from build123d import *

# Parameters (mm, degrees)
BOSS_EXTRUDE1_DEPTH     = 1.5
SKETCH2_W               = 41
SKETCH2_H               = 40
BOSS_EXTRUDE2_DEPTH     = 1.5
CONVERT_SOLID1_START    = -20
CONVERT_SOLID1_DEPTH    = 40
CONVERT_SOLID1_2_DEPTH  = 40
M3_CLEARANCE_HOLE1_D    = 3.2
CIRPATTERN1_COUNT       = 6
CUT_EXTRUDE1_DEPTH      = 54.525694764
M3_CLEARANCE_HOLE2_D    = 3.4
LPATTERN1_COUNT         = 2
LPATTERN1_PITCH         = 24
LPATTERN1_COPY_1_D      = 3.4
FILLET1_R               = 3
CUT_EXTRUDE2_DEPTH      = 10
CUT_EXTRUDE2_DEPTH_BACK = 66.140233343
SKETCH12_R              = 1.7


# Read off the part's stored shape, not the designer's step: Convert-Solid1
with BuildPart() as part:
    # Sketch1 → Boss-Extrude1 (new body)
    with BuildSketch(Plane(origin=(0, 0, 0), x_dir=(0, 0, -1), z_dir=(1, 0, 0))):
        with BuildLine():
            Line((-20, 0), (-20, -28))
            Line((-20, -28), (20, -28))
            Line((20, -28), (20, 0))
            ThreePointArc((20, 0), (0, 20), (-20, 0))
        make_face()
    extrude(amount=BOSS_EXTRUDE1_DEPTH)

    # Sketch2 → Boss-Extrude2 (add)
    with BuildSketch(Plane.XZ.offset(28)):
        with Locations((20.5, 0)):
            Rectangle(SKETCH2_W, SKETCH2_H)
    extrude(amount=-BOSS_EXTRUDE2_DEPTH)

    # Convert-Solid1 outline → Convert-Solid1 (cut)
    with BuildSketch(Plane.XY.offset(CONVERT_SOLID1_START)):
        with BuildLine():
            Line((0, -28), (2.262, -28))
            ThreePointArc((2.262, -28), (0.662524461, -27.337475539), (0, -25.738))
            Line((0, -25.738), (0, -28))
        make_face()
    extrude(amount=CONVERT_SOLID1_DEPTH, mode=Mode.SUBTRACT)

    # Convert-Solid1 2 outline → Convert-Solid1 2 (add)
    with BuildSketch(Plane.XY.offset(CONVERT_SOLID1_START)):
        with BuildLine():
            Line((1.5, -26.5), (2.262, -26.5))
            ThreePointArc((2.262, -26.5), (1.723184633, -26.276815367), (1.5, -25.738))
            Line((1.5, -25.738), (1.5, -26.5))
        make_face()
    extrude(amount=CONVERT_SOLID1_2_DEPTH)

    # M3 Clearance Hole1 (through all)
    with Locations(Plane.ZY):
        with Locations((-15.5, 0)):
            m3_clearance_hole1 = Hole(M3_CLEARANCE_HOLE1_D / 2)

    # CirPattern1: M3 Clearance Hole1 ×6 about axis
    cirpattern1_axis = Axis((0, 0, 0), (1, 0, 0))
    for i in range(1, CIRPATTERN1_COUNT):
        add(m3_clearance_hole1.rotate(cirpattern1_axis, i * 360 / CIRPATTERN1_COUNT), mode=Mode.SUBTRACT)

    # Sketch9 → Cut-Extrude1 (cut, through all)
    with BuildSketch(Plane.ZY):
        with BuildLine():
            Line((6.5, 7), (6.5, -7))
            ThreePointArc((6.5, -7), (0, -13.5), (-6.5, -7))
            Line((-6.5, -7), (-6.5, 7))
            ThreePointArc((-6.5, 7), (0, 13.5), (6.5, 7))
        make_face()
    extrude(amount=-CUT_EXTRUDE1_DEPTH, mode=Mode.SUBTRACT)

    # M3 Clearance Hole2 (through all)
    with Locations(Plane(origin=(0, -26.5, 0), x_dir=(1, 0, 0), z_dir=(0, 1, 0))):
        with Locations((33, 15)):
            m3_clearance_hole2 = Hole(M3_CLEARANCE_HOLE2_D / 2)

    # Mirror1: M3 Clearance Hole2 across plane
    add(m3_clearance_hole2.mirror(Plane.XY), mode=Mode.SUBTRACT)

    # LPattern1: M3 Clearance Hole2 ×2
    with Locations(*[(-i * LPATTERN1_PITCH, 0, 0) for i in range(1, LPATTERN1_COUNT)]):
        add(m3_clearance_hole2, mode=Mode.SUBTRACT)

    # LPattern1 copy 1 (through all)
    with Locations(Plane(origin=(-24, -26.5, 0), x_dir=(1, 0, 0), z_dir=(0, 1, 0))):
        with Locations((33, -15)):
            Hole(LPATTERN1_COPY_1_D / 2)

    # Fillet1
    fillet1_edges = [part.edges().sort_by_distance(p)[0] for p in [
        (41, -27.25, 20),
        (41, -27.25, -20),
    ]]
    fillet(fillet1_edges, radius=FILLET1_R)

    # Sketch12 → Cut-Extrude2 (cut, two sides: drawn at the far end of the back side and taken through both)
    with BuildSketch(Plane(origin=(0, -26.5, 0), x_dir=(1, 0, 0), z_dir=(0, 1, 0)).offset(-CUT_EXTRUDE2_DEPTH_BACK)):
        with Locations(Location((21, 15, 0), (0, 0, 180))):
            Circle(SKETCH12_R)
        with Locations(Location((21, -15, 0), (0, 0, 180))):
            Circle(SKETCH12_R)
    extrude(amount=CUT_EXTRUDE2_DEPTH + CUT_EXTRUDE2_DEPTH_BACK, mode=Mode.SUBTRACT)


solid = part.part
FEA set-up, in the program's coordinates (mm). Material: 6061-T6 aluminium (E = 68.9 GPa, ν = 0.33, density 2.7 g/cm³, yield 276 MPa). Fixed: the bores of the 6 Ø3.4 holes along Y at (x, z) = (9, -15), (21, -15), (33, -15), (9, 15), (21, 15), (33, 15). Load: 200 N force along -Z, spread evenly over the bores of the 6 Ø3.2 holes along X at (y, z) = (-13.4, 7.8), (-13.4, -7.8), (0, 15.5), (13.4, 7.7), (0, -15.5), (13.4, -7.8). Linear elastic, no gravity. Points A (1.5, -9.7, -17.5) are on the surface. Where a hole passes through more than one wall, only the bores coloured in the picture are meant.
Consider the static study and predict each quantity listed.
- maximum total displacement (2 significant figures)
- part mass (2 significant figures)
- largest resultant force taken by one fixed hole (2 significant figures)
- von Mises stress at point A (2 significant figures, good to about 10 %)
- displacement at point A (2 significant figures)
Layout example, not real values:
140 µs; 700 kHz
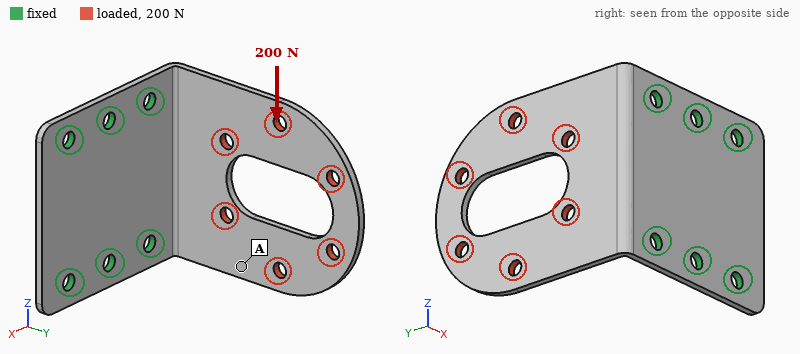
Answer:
0.24 mm; 12 g; 210 N; 22 MPa; 0.16 mm
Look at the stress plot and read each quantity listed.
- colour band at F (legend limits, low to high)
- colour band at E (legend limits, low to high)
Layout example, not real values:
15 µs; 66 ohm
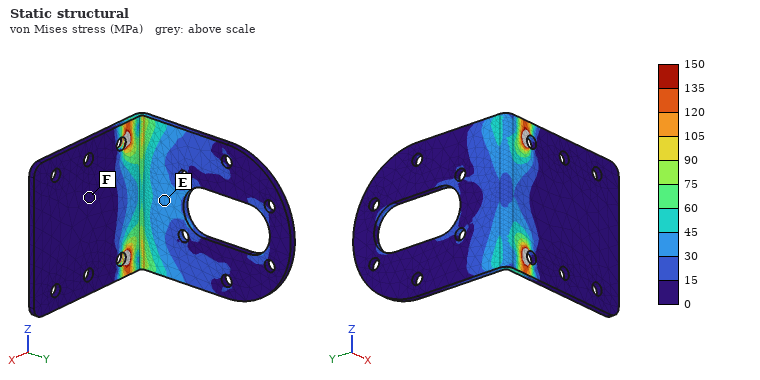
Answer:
0 to 15 MPa; 30 to 45 MPa
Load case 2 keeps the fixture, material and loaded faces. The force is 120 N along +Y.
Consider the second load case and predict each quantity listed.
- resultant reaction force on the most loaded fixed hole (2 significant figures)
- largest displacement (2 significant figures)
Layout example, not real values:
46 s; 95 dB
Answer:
68 N; 0.23 mm
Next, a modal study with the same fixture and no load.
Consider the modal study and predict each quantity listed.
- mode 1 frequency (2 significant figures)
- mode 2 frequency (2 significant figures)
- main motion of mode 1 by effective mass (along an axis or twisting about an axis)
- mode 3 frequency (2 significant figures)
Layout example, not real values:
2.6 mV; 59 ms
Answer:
570 Hz; 1500 Hz; along X; 2800 Hz
